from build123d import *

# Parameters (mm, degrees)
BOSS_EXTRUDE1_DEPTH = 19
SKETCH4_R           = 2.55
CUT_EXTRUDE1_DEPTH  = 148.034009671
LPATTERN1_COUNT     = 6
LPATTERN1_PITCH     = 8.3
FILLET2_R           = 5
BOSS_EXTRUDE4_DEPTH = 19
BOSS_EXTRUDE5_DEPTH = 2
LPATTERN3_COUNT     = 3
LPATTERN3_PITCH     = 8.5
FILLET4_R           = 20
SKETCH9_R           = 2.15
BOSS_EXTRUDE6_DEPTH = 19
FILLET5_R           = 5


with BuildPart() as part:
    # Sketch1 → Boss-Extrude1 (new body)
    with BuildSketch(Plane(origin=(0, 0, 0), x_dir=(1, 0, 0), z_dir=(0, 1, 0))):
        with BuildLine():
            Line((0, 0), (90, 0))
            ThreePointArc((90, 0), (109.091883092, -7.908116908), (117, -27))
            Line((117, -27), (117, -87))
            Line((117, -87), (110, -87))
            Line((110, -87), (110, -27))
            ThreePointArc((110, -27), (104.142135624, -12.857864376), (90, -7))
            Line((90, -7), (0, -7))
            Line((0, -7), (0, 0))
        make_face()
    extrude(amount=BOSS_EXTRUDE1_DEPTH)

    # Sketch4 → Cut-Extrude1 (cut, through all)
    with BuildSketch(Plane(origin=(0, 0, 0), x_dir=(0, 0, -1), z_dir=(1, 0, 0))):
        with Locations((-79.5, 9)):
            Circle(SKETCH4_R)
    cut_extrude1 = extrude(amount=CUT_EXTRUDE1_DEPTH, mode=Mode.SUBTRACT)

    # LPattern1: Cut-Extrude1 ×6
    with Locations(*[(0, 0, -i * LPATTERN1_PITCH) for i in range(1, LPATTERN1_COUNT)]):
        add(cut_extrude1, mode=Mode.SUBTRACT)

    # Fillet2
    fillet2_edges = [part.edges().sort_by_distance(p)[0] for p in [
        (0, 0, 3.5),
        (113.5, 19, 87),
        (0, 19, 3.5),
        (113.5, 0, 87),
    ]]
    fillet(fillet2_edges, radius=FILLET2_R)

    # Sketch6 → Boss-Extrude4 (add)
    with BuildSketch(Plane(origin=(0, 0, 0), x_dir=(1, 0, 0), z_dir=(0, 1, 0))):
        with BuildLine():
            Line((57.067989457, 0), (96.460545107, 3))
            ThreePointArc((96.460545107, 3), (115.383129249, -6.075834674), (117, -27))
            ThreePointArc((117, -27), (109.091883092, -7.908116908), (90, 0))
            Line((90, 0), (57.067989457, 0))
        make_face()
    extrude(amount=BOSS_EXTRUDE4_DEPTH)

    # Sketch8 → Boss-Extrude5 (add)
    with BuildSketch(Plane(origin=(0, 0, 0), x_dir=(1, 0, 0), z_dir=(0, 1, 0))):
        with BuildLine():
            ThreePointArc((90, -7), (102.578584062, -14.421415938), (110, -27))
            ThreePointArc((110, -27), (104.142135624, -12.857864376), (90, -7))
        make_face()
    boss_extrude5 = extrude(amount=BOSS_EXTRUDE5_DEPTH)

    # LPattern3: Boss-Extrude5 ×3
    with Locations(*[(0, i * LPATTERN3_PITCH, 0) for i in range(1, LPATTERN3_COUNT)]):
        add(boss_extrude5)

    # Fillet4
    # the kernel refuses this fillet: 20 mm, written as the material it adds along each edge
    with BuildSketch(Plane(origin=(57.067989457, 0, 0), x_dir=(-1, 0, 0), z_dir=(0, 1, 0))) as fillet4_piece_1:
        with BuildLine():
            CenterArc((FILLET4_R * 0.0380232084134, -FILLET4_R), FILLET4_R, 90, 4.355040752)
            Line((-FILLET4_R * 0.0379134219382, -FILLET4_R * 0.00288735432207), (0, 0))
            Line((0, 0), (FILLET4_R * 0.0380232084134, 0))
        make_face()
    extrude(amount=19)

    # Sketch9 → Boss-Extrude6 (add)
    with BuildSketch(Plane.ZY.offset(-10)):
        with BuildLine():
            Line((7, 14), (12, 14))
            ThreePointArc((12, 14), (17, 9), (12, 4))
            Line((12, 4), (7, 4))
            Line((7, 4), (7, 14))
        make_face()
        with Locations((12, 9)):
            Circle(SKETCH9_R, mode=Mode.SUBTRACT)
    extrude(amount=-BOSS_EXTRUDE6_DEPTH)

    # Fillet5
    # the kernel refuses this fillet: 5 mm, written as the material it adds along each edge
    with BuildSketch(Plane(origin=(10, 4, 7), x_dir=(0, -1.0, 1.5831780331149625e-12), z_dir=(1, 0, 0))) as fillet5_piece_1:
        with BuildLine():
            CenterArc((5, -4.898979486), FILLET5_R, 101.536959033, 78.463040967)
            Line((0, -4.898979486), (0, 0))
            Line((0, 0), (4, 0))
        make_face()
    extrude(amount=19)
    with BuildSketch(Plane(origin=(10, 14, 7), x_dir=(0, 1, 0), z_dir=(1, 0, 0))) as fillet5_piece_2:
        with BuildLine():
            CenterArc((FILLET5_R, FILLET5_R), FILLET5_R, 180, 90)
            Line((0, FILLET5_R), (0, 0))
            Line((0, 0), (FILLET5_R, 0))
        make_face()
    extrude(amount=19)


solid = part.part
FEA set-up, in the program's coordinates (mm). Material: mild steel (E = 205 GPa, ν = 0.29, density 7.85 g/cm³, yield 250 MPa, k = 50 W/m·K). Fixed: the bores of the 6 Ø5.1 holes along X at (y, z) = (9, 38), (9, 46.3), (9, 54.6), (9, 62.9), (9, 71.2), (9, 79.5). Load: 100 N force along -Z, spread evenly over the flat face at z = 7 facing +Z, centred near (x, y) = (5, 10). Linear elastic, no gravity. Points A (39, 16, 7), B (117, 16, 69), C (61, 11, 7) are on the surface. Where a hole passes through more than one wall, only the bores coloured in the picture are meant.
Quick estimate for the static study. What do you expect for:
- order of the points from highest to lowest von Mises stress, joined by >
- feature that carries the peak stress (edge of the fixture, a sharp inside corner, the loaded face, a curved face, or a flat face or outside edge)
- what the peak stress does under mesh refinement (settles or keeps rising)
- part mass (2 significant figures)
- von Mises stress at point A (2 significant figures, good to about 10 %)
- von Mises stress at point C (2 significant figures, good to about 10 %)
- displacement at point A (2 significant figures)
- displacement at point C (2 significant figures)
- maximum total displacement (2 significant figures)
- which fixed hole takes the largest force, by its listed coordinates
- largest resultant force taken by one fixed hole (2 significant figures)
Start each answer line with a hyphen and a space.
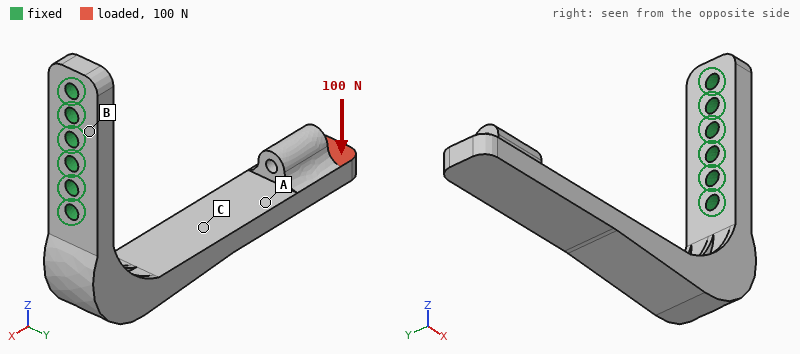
- C > A > B
- edge of the fixture
- keeps rising
- 240 g
- 22 MPa
- 33 MPa
- 0.19 mm
- 0.12 mm
- 0.36 mm
- (9, 38)
- 310 N
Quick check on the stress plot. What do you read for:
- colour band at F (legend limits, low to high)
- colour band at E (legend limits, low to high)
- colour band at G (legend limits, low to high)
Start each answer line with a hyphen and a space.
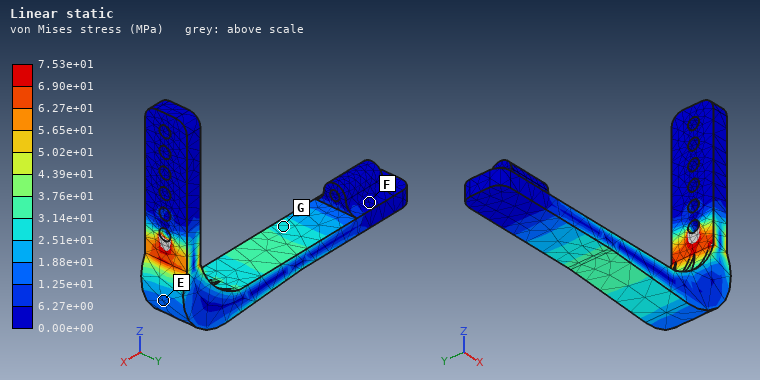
- 0.00e+00 to 6.27e+00 MPa
- 1.25e+01 to 1.88e+01 MPa
- 2.51e+01 to 3.14e+01 MPa
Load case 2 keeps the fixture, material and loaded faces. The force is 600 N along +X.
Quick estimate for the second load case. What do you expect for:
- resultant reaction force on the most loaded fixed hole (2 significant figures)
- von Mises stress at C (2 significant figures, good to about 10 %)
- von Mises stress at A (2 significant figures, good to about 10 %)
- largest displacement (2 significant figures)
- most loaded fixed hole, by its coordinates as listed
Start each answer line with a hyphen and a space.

- 1.0 kN
- 17 MPa
- 18 MPa
- 0.16 mm
- (9, 38)
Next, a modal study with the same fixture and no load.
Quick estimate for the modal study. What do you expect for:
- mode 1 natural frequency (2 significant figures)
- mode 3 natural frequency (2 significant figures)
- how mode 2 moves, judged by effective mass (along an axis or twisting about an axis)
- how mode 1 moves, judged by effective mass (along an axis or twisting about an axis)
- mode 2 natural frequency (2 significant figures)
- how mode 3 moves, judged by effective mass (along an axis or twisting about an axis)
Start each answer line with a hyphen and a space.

- 400 Hz
- 1600 Hz
- along Y
- along Z
- 530 Hz
- along X
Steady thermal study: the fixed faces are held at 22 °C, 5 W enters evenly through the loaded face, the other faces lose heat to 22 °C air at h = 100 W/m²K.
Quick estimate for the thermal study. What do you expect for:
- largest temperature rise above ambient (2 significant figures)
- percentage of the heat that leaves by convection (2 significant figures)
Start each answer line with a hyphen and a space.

- 21 K
- 96 %
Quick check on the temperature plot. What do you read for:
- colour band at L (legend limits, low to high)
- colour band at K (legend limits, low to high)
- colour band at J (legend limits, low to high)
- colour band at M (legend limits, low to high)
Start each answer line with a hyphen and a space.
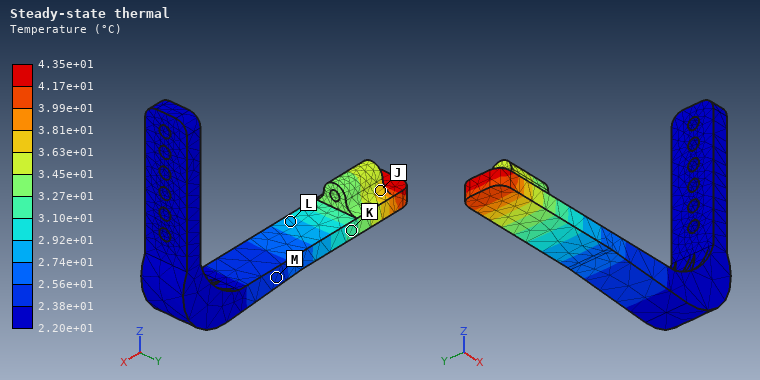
- 2.74e+01 to 2.92e+01 °C
- 3.10e+01 to 3.27e+01 °C
- 3.63e+01 to 3.81e+01 °C
- 2.38e+01 to 2.56e+01 °C
